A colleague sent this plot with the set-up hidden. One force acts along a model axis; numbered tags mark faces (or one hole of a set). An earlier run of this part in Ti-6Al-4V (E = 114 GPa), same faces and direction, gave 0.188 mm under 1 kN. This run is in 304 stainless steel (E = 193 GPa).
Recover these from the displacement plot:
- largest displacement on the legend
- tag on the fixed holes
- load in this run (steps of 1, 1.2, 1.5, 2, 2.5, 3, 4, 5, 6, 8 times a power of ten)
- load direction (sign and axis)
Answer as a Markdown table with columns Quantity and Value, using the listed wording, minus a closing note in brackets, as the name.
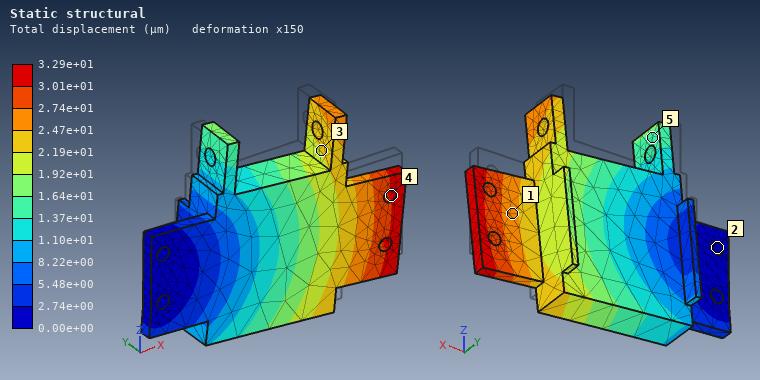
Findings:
| Quantity | Value |
|---|---|
| largest displacement on the legend | 3.29e+01 µm |
| tag on the fixed holes | 2 |
| load in this run | 300 N |
| load direction | -Z |
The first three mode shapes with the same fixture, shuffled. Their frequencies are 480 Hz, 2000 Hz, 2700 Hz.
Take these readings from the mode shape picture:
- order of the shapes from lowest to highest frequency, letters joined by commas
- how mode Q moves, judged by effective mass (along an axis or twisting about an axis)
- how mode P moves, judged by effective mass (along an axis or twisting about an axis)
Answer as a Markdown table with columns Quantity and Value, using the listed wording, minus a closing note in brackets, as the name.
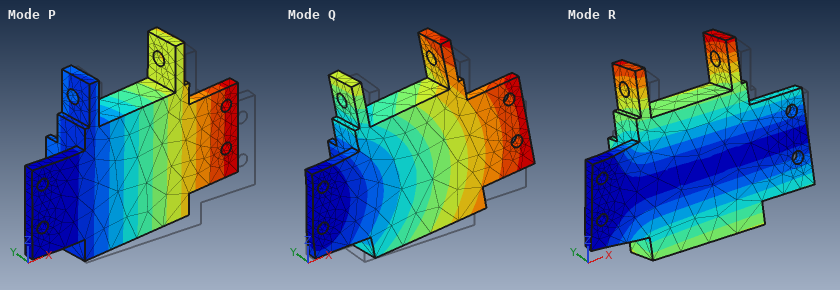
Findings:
| Quantity | Value |
|---|---|
| order of the shapes from lowest to highest frequency, letters joined by commas | P, R, Q |
| how mode Q moves, judged by effective mass | along Z |
| how mode P moves, judged by effective mass | along Y |
